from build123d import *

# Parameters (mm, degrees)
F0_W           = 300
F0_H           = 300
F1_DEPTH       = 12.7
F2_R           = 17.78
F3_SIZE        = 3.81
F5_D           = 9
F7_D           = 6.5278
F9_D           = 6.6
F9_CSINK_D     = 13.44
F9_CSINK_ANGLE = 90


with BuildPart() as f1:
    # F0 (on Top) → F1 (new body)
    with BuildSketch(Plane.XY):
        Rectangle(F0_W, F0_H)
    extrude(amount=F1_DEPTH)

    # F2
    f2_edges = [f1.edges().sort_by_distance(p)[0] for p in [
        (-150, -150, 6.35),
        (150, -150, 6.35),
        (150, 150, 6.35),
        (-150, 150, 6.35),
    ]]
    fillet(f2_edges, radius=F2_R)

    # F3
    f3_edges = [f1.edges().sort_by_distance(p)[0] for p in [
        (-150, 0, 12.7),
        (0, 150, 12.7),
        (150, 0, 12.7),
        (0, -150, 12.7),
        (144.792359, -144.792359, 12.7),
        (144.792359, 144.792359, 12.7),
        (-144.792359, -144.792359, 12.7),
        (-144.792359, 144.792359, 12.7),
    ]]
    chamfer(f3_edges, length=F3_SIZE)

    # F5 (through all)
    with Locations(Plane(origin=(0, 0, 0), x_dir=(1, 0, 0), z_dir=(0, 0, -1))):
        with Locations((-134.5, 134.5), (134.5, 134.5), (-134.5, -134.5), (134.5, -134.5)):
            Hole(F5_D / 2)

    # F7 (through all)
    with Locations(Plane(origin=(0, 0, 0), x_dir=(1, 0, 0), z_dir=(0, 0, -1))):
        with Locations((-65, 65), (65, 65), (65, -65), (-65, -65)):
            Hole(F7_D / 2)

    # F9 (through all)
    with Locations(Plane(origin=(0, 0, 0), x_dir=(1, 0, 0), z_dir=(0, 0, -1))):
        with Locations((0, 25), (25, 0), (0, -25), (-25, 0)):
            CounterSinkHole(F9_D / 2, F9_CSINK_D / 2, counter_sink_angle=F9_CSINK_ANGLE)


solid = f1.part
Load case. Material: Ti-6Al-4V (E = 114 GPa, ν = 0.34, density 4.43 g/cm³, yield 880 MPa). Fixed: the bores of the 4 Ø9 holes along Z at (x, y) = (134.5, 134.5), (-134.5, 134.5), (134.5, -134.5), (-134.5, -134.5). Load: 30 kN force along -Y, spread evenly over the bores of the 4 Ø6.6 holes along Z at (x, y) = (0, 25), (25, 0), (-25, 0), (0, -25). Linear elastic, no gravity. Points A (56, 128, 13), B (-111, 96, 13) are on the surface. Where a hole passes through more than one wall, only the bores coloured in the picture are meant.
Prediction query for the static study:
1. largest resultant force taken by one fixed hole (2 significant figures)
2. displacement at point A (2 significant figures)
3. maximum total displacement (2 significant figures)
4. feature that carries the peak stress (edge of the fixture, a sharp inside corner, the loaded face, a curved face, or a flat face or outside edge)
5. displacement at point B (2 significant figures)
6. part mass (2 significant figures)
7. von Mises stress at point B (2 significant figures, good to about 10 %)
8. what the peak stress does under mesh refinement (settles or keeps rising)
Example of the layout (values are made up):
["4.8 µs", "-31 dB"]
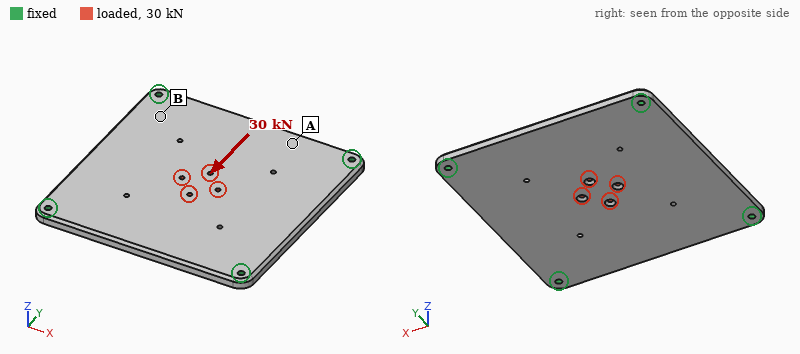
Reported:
["8.5 kN", "15 µm", "27 µm", "a sharp inside corner", "7.4 µm", "5.0 kg", "11 MPa", "keeps rising"]
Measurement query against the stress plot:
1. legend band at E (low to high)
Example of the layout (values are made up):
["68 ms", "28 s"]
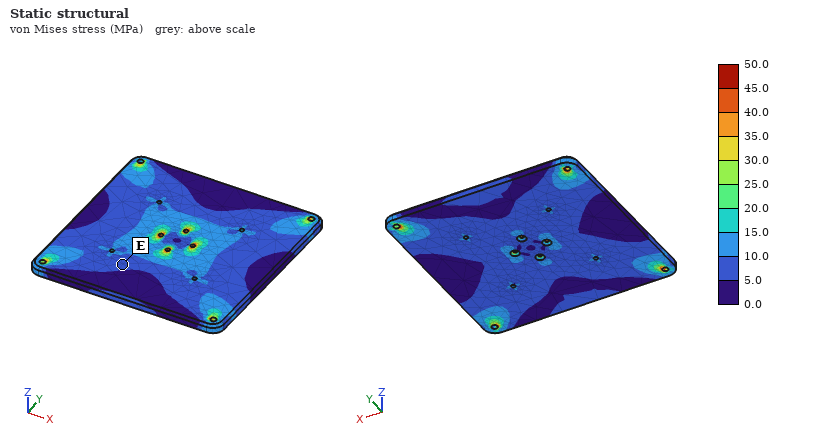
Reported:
["5.0 to 10.0 MPa"]
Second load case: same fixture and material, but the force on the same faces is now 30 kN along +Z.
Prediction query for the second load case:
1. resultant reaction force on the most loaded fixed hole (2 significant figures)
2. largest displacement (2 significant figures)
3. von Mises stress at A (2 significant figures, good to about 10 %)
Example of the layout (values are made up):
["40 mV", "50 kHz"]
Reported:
["7.5 kN", "1.7 mm", "52 MPa"]
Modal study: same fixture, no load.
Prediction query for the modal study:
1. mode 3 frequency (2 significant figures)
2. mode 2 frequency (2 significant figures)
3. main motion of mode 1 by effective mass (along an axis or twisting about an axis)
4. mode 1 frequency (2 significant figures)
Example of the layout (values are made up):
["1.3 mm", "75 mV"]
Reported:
["950 Hz", "950 Hz", "along Z", "530 Hz"]
